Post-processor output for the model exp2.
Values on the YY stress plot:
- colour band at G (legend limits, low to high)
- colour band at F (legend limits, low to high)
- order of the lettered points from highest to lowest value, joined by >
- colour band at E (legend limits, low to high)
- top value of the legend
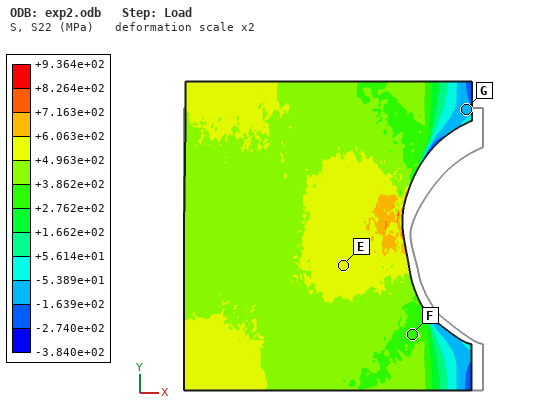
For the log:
-1.639e+02 to -5.389e+01 MPa
+2.762e+02 to +3.862e+02 MPa
E > F > G
+4.963e+02 to +6.063e+02 MPa
+9.364e+02 MPa
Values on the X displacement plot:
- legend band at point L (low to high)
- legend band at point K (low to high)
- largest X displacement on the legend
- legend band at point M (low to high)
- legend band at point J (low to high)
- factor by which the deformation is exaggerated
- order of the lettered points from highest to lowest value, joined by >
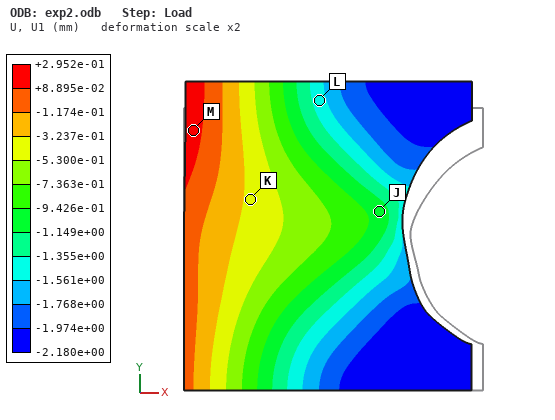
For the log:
-1.561e+00 to -1.355e+00 mm
-5.300e-01 to -3.237e-01 mm
+2.952e-01 mm
+8.895e-02 to +2.952e-01 mm
-1.149e+00 to -9.426e-01 mm
2
M > K > J > L
